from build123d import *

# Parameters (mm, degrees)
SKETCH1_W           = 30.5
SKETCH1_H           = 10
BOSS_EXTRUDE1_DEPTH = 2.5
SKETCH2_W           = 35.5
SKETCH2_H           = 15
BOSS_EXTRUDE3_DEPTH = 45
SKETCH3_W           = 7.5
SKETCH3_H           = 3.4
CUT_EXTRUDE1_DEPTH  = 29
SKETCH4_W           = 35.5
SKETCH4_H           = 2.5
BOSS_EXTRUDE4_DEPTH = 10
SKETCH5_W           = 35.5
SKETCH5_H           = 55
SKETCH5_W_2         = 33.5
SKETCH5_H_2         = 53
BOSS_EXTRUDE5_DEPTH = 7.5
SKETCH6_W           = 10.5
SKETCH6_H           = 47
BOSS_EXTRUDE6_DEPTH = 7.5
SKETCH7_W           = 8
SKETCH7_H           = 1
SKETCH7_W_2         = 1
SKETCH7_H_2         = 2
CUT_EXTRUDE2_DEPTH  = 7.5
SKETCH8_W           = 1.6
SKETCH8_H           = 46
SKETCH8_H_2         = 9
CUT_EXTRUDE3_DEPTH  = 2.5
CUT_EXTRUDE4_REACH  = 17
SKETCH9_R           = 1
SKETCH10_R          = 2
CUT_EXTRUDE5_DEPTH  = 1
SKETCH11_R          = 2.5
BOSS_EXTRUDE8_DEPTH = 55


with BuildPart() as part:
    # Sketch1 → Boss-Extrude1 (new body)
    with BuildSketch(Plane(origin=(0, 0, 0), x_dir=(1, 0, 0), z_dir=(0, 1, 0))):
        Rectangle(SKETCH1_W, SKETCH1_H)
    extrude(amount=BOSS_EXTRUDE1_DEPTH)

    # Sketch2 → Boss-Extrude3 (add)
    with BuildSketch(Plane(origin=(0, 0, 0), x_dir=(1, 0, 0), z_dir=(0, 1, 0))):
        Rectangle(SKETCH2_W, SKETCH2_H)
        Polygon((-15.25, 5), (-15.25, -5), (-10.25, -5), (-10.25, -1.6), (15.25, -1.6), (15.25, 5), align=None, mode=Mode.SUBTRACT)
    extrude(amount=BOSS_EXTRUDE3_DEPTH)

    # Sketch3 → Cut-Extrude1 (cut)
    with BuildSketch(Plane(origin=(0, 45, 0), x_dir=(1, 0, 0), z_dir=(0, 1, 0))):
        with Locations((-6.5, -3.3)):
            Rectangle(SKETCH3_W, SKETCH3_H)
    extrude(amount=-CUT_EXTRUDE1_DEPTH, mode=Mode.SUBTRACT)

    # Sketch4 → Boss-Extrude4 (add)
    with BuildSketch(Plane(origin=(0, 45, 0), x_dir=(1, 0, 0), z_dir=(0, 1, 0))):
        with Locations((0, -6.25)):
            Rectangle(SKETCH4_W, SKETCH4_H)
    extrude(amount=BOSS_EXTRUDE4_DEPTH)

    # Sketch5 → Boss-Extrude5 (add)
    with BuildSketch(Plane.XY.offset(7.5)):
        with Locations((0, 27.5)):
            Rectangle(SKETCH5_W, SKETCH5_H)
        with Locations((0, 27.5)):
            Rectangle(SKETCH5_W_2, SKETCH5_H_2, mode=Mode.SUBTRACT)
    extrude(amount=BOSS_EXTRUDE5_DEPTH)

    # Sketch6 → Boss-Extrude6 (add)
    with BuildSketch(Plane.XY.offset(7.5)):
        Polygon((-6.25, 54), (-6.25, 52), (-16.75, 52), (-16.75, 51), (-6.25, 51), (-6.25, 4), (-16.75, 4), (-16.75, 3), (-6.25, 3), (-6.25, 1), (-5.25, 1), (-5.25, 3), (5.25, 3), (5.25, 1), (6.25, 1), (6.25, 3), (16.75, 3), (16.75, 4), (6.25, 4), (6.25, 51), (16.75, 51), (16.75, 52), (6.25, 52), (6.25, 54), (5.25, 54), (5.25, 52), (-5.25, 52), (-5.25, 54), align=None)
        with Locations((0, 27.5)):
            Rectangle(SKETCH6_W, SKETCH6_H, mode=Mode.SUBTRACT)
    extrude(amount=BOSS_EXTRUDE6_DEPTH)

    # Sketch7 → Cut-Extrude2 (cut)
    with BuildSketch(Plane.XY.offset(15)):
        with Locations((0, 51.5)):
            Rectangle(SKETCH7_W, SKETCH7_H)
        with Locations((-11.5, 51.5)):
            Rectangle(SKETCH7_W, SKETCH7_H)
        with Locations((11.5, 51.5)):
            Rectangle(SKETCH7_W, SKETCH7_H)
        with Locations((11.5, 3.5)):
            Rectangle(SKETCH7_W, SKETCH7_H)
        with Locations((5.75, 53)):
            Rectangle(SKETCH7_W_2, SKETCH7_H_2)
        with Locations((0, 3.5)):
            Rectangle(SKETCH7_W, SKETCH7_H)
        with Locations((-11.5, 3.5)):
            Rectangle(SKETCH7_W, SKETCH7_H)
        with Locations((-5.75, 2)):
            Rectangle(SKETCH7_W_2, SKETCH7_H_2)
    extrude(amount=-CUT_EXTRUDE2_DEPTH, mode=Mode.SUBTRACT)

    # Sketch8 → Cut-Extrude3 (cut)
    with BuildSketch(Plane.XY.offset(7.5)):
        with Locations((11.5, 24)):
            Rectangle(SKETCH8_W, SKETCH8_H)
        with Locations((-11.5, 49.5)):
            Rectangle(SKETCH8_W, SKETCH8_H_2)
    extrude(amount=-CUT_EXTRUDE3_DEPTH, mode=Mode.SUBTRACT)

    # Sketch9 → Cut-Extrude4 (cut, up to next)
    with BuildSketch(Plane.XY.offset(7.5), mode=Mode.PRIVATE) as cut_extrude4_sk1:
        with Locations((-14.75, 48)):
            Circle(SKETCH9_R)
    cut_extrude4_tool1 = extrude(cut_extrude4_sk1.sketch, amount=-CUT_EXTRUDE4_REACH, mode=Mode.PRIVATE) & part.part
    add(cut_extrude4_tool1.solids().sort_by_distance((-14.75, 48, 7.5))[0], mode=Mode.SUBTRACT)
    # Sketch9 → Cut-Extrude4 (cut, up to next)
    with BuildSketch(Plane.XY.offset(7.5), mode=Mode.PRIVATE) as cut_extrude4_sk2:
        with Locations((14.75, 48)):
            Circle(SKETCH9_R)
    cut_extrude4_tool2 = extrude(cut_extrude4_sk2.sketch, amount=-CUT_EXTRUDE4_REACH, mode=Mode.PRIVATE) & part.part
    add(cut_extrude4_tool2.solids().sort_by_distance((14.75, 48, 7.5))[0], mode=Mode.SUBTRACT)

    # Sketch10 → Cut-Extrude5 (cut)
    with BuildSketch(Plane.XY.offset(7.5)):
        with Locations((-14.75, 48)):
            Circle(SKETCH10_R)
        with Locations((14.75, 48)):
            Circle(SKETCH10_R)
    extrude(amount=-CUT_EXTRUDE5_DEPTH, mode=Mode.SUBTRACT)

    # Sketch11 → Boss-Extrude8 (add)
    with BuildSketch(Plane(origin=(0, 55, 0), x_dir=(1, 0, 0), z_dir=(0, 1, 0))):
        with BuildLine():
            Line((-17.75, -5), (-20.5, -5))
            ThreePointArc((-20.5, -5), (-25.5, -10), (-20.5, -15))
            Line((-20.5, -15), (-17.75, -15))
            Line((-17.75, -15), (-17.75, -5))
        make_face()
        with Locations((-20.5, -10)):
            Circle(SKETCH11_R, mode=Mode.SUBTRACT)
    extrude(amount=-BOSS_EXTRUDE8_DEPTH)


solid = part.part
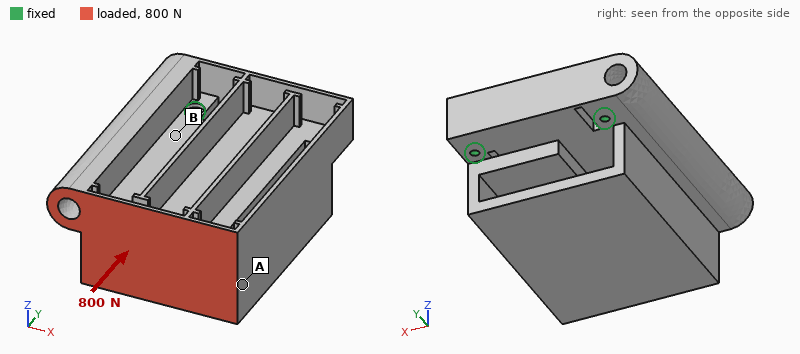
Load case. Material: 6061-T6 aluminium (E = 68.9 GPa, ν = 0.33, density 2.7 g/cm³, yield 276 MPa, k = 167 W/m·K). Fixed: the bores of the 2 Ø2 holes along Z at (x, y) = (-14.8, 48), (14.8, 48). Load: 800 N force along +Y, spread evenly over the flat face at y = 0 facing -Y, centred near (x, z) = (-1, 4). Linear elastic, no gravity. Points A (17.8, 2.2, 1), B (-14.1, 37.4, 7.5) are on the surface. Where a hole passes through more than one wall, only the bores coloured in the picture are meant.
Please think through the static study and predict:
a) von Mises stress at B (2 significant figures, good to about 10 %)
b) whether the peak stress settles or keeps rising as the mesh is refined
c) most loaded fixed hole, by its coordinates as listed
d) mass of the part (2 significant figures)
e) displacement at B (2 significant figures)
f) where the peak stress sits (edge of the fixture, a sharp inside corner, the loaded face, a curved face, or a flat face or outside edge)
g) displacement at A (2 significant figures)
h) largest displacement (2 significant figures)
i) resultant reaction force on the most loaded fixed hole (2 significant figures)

10 MPa
keeps rising
(-14.8, 48)
52 g
0.031 mm
edge of the fixture
0.15 mm
0.16 mm
430 N
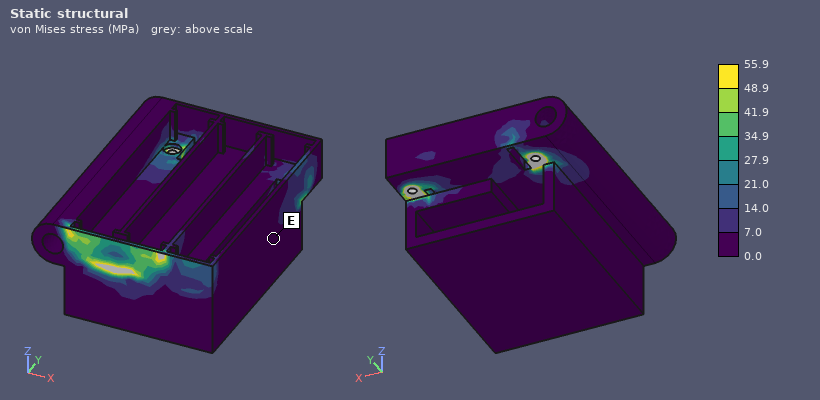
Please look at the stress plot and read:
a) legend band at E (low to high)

0.0 to 7.0 MPa
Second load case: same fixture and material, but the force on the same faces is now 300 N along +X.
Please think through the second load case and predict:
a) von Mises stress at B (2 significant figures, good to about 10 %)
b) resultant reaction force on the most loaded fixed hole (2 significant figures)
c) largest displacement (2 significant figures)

8.8 MPa
510 N
23 µm
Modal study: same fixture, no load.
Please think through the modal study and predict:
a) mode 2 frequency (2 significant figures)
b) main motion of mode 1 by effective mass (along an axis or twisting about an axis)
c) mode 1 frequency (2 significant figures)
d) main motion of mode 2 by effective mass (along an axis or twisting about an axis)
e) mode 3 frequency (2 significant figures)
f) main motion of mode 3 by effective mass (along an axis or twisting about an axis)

3700 Hz
along Z
510 Hz
along X
4300 Hz
along X
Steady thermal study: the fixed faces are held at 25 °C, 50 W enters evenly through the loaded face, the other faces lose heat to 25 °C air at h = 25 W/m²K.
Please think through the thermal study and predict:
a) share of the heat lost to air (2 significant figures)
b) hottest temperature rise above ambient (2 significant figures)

29 %
67 K
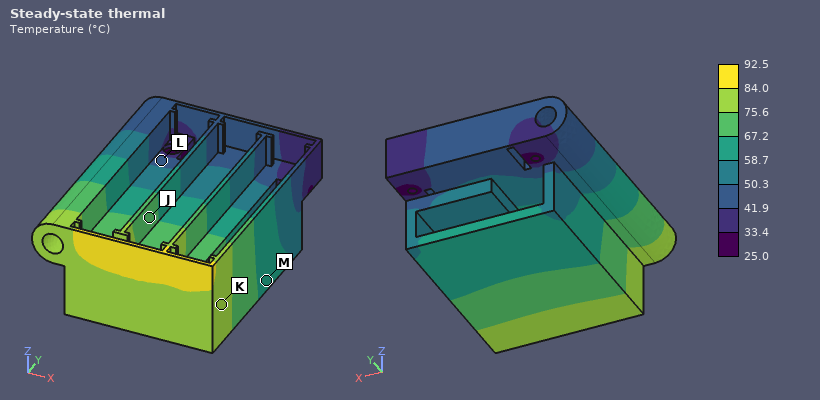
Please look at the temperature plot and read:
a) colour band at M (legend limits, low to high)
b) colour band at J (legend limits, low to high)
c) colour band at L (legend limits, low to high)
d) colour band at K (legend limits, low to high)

58.7 to 67.2 °C
67.2 to 75.6 °C
41.9 to 50.3 °C
75.6 to 84.0 °C
